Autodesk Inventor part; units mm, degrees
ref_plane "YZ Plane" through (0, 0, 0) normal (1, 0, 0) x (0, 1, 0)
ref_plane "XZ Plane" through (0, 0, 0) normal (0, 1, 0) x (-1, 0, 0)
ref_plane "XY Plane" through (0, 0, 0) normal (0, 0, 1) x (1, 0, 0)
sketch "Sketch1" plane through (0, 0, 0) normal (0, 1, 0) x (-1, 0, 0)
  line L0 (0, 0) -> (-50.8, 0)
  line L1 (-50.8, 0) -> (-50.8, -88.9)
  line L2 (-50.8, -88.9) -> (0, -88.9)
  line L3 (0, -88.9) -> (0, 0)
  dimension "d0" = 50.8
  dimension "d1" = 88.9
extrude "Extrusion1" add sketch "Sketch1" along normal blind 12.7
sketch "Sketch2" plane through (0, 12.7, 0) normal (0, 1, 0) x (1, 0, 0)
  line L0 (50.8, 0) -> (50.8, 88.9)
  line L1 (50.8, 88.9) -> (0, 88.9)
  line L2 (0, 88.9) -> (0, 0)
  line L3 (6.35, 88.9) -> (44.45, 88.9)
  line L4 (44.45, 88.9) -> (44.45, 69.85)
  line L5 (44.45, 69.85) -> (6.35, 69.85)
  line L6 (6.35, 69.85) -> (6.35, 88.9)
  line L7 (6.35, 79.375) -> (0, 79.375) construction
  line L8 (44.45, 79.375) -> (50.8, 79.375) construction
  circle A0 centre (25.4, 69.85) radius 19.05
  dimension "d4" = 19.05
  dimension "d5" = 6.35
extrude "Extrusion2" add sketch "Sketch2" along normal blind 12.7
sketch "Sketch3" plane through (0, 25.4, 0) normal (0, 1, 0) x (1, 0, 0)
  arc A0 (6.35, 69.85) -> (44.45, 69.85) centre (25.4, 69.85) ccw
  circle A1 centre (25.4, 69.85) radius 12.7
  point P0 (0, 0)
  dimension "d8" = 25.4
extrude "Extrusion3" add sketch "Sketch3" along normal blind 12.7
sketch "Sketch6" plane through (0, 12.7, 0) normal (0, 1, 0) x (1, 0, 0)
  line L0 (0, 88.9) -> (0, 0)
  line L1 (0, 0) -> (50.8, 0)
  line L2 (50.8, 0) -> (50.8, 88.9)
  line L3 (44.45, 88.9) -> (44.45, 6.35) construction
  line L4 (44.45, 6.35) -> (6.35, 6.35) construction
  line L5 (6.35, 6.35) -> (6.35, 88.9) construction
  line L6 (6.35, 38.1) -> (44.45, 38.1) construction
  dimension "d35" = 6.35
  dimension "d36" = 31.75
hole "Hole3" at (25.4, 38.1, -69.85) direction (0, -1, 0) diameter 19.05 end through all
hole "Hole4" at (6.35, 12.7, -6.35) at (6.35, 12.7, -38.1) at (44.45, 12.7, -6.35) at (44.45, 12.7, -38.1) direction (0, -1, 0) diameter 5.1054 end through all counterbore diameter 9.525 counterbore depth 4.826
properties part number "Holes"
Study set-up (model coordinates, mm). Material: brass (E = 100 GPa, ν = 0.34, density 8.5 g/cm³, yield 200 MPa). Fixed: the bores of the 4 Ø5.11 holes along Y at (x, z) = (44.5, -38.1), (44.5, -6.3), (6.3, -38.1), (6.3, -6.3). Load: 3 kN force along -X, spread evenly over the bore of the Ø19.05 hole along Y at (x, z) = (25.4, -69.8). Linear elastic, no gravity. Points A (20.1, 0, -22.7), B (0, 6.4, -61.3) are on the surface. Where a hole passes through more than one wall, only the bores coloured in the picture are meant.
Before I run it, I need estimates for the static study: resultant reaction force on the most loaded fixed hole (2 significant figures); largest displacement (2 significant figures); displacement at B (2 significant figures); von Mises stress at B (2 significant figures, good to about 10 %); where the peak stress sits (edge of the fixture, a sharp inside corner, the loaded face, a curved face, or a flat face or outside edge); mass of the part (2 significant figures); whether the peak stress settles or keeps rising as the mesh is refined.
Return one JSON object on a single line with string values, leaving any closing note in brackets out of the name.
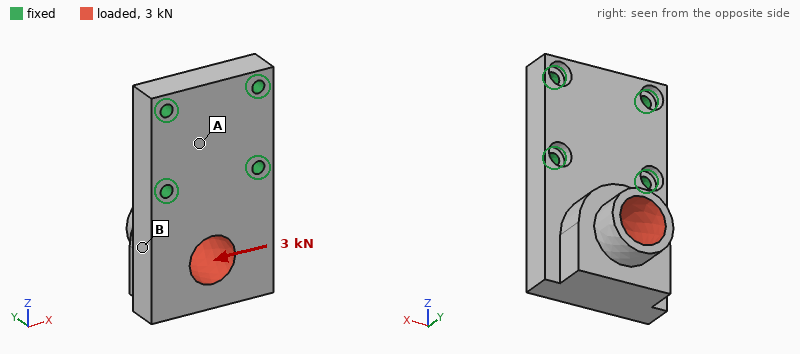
{"resultant reaction force on the most loaded fixed hole": "2.9 kN", "largest displacement": "25 µm", "displacement at B": "10 µm", "von Mises stress at B": "9.1 MPa", "where the peak stress sits": "edge of the fixture", "mass of the part": "570 g", "whether the peak stress settles or keeps rising as the mesh is refined": "keeps rising"}
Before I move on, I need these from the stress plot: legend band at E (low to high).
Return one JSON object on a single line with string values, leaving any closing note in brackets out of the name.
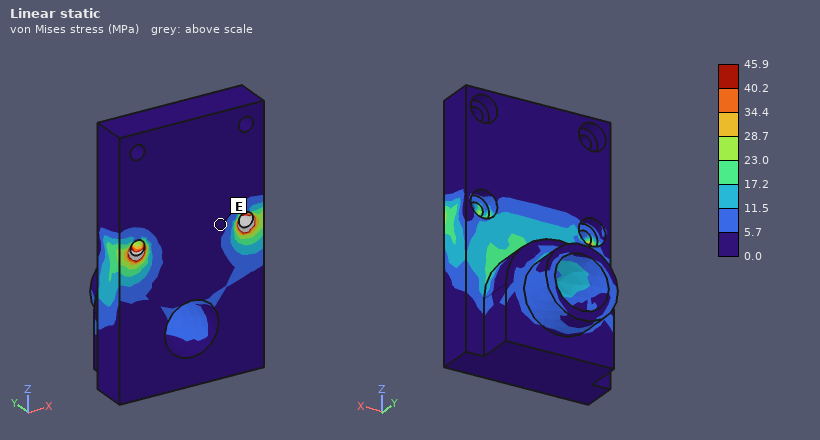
{"legend band at E": "0.0 to 5.7 MPa"}
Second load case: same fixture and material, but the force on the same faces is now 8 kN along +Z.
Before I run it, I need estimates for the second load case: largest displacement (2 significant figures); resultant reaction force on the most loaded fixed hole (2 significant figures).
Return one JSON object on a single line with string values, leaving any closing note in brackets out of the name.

{"largest displacement": "0.19 mm", "resultant reaction force on the most loaded fixed hole": "2.4 kN"}
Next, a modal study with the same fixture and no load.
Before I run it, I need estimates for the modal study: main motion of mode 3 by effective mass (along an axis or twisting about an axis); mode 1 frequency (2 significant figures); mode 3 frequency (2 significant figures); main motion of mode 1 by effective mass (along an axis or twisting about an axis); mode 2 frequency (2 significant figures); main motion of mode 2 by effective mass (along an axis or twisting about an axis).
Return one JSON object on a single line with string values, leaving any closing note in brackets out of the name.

{"main motion of mode 3 by effective mass": "along X", "mode 1 frequency": "1600 Hz", "mode 3 frequency": "4900 Hz", "main motion of mode 1 by effective mass": "along Y", "mode 2 frequency": "4400 Hz", "main motion of mode 2 by effective mass": "along X"}
